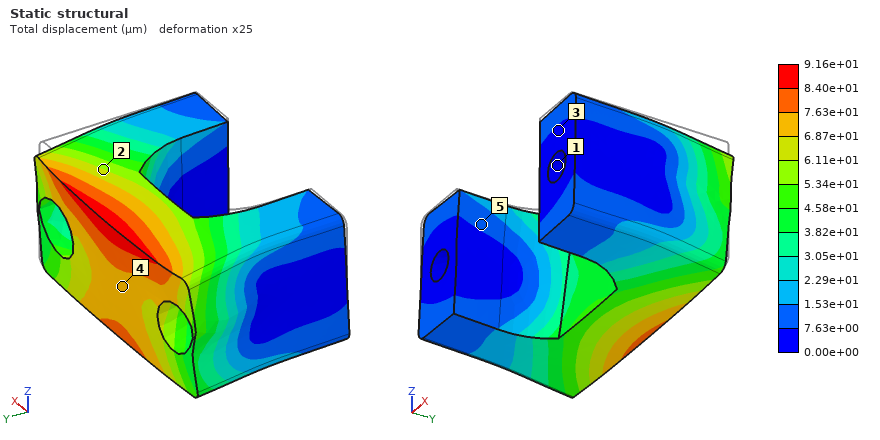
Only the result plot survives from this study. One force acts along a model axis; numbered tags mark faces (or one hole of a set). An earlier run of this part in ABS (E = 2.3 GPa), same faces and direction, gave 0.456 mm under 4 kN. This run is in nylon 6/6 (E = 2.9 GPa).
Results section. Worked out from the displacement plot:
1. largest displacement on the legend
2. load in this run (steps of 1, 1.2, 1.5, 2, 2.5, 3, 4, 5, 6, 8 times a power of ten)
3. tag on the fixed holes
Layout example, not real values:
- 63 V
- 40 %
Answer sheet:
- 9.16e+01 µm
- 1 kN
- 1
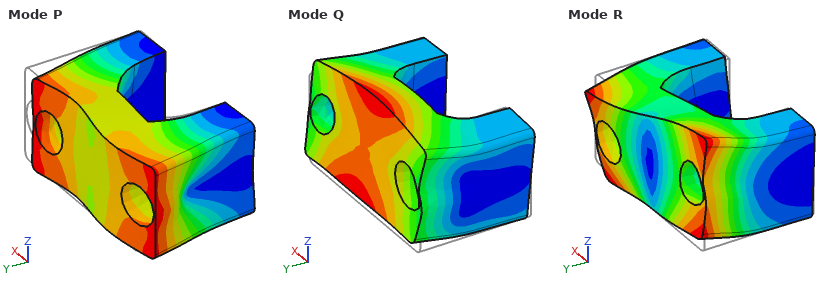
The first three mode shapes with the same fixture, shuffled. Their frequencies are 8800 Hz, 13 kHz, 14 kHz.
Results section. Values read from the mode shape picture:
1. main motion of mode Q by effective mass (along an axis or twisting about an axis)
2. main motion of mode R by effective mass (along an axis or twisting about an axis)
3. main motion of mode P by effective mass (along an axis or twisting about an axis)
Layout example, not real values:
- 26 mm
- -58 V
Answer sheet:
- along Z
- twisting about Y
- along X
